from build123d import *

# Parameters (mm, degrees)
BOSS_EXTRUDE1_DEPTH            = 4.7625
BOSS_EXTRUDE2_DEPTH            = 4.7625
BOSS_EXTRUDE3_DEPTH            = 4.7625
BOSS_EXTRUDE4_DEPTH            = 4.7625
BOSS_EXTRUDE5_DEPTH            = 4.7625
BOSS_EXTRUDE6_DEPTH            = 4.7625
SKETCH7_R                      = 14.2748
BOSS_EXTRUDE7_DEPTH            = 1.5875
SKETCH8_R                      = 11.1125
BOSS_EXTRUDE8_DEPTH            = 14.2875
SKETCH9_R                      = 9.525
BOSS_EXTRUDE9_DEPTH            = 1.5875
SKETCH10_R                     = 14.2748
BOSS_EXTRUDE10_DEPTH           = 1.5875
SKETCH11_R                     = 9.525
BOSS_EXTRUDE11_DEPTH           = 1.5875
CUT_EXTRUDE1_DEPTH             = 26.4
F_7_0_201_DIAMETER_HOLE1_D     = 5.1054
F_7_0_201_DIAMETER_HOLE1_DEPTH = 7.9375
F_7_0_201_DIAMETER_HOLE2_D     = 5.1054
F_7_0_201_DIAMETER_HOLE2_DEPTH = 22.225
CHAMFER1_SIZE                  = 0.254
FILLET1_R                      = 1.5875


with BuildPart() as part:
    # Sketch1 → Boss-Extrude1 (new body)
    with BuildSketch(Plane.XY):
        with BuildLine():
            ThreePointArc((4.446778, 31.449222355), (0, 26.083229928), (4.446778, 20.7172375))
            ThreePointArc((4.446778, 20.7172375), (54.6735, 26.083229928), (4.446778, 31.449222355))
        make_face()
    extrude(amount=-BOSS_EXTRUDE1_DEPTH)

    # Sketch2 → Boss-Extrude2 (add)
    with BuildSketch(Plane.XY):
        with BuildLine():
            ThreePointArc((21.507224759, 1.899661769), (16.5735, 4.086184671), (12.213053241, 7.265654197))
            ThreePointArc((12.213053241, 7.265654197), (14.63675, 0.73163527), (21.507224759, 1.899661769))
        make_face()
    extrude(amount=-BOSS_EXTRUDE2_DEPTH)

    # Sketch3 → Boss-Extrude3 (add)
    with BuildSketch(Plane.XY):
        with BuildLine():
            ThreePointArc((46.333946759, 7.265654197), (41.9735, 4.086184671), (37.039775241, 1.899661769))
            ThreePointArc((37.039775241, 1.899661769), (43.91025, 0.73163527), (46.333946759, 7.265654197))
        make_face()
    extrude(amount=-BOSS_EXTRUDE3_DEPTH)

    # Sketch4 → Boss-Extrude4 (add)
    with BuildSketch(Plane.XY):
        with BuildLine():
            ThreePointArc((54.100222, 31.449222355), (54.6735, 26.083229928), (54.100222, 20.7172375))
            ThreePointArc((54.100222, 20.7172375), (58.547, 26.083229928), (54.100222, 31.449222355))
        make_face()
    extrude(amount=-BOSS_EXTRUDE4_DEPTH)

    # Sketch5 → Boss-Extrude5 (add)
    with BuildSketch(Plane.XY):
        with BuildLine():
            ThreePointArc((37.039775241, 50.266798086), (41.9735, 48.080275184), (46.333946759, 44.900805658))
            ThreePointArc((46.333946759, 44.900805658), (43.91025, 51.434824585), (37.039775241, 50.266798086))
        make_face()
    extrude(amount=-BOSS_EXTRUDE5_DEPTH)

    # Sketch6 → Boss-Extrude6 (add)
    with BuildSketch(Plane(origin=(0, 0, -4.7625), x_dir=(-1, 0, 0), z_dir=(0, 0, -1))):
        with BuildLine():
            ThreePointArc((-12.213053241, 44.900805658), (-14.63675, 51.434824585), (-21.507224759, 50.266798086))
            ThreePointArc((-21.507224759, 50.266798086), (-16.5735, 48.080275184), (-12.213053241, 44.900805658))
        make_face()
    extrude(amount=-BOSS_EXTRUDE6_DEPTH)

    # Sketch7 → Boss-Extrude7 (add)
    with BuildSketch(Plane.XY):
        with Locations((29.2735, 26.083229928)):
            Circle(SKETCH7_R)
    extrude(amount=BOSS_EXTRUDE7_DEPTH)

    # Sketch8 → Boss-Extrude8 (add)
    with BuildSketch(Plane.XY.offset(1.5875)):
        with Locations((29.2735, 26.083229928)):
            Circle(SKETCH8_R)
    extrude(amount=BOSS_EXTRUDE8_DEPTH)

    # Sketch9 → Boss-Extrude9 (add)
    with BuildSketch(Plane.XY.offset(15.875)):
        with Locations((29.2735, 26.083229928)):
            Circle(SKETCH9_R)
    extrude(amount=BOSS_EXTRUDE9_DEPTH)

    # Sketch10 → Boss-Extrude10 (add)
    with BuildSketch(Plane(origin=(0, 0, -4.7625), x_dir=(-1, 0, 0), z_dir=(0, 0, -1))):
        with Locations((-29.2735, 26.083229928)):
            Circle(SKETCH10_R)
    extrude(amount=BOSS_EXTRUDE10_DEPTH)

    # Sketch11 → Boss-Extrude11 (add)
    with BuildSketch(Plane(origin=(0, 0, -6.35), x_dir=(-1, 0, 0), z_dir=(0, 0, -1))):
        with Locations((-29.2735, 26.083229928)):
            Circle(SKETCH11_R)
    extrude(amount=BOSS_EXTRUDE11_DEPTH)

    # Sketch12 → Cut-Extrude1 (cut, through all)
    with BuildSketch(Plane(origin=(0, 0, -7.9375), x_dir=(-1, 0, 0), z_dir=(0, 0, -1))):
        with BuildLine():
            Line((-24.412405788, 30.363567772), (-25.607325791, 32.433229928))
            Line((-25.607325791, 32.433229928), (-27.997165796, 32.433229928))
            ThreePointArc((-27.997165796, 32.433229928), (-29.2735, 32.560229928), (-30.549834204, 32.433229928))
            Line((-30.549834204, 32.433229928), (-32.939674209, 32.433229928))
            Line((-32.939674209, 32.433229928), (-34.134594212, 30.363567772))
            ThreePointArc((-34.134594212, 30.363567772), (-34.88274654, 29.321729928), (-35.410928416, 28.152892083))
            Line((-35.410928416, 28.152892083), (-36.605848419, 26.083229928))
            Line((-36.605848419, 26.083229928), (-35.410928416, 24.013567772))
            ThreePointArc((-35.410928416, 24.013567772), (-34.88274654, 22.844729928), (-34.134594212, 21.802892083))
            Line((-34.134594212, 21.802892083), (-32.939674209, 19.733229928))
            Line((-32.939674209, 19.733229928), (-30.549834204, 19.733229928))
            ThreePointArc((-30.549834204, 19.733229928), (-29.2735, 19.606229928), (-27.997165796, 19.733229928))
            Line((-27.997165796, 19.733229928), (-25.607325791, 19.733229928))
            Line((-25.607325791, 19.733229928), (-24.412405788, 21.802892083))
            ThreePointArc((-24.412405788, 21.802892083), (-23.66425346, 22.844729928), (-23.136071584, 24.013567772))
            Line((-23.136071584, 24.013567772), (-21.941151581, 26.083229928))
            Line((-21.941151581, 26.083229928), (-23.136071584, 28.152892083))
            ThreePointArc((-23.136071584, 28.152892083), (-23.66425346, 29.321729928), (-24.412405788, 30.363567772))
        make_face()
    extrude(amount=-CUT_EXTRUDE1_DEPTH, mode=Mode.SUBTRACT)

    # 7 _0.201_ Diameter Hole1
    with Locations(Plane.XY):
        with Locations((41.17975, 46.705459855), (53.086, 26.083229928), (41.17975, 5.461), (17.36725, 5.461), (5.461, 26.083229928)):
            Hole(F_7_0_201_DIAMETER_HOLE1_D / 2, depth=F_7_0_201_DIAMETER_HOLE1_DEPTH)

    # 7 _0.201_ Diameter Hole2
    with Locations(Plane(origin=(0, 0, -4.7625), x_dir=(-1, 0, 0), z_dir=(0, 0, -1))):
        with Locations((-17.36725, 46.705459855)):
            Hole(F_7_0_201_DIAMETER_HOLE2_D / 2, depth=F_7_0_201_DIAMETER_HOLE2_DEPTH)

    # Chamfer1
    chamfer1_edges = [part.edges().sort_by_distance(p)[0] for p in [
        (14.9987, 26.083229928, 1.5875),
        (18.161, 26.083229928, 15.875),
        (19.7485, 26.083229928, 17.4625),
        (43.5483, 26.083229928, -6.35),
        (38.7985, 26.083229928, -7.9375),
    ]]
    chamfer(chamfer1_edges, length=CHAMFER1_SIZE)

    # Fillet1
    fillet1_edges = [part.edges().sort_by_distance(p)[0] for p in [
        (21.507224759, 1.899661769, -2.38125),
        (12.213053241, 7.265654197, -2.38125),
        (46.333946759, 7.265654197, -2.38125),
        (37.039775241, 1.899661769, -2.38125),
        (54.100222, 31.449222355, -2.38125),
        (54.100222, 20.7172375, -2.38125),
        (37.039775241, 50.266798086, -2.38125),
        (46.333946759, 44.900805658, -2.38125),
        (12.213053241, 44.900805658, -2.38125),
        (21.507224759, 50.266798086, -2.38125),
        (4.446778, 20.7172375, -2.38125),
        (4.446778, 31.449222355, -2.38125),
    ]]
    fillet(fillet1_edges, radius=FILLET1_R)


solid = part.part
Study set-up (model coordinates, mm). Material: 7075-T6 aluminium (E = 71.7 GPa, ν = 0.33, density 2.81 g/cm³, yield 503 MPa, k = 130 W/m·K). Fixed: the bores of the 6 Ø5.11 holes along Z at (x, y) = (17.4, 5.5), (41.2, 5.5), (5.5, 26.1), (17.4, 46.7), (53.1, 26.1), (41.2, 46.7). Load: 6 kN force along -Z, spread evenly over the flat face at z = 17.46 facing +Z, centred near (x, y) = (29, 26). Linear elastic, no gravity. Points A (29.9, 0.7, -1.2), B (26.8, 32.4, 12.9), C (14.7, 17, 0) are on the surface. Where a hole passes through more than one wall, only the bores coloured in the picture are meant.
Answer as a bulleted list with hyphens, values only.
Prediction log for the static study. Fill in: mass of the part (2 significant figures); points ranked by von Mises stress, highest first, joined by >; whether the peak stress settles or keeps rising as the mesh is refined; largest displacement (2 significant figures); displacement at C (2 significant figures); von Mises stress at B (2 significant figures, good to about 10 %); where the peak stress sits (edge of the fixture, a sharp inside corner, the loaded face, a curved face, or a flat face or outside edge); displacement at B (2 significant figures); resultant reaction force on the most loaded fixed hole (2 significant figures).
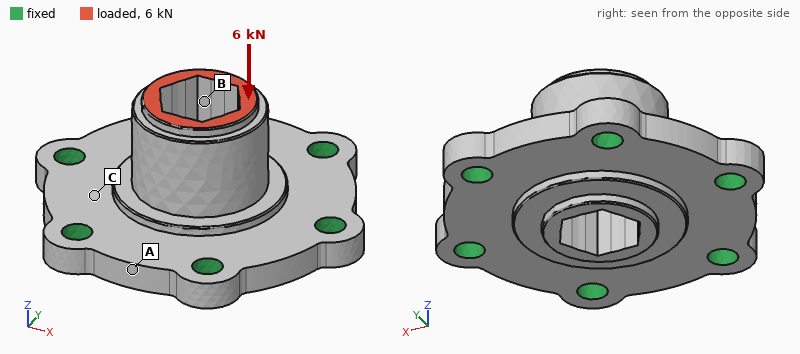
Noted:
- 42 g
- B > C > A
- keeps rising
- 29 µm
- 11 µm
- 45 MPa
- edge of the fixture
- 26 µm
- 1.0 kN
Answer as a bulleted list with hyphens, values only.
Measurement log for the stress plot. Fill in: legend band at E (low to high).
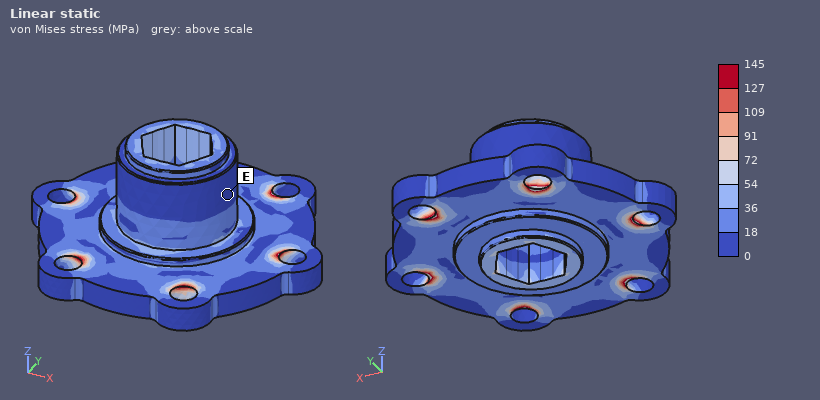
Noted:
- 0 to 18 MPa
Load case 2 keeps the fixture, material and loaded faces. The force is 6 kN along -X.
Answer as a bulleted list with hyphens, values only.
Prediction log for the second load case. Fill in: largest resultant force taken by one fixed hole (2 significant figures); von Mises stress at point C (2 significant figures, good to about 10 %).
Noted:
- 2.6 kN
- 55 MPa
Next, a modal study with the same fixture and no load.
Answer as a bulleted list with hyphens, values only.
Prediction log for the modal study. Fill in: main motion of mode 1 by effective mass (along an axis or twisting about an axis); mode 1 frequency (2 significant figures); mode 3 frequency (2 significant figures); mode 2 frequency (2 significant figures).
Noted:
- along Z
- 17 kHz
- 18 kHz
- 18 kHz
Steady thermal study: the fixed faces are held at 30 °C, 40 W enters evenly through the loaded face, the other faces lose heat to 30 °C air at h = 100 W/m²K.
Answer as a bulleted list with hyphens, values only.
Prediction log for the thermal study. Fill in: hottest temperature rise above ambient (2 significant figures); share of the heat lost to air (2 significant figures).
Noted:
- 31 K
- 14 %
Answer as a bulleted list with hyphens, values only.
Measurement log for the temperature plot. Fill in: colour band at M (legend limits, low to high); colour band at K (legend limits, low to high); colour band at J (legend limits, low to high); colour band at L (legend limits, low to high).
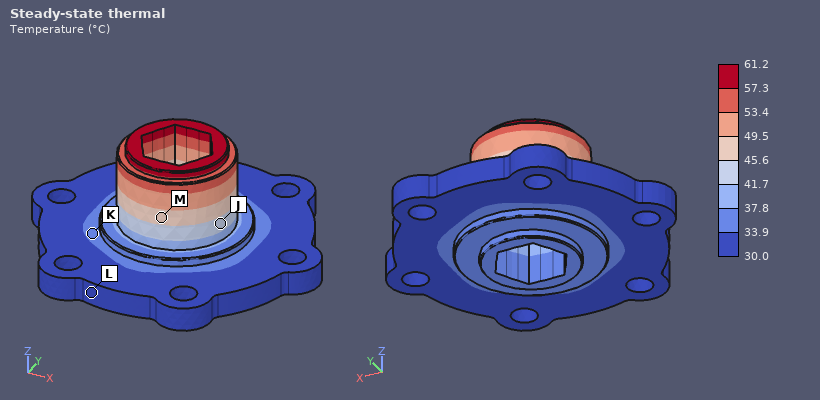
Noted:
- 45.6 to 49.5 °C
- 33.9 to 37.8 °C
- 41.7 to 45.6 °C
- 30.0 to 33.9 °C
